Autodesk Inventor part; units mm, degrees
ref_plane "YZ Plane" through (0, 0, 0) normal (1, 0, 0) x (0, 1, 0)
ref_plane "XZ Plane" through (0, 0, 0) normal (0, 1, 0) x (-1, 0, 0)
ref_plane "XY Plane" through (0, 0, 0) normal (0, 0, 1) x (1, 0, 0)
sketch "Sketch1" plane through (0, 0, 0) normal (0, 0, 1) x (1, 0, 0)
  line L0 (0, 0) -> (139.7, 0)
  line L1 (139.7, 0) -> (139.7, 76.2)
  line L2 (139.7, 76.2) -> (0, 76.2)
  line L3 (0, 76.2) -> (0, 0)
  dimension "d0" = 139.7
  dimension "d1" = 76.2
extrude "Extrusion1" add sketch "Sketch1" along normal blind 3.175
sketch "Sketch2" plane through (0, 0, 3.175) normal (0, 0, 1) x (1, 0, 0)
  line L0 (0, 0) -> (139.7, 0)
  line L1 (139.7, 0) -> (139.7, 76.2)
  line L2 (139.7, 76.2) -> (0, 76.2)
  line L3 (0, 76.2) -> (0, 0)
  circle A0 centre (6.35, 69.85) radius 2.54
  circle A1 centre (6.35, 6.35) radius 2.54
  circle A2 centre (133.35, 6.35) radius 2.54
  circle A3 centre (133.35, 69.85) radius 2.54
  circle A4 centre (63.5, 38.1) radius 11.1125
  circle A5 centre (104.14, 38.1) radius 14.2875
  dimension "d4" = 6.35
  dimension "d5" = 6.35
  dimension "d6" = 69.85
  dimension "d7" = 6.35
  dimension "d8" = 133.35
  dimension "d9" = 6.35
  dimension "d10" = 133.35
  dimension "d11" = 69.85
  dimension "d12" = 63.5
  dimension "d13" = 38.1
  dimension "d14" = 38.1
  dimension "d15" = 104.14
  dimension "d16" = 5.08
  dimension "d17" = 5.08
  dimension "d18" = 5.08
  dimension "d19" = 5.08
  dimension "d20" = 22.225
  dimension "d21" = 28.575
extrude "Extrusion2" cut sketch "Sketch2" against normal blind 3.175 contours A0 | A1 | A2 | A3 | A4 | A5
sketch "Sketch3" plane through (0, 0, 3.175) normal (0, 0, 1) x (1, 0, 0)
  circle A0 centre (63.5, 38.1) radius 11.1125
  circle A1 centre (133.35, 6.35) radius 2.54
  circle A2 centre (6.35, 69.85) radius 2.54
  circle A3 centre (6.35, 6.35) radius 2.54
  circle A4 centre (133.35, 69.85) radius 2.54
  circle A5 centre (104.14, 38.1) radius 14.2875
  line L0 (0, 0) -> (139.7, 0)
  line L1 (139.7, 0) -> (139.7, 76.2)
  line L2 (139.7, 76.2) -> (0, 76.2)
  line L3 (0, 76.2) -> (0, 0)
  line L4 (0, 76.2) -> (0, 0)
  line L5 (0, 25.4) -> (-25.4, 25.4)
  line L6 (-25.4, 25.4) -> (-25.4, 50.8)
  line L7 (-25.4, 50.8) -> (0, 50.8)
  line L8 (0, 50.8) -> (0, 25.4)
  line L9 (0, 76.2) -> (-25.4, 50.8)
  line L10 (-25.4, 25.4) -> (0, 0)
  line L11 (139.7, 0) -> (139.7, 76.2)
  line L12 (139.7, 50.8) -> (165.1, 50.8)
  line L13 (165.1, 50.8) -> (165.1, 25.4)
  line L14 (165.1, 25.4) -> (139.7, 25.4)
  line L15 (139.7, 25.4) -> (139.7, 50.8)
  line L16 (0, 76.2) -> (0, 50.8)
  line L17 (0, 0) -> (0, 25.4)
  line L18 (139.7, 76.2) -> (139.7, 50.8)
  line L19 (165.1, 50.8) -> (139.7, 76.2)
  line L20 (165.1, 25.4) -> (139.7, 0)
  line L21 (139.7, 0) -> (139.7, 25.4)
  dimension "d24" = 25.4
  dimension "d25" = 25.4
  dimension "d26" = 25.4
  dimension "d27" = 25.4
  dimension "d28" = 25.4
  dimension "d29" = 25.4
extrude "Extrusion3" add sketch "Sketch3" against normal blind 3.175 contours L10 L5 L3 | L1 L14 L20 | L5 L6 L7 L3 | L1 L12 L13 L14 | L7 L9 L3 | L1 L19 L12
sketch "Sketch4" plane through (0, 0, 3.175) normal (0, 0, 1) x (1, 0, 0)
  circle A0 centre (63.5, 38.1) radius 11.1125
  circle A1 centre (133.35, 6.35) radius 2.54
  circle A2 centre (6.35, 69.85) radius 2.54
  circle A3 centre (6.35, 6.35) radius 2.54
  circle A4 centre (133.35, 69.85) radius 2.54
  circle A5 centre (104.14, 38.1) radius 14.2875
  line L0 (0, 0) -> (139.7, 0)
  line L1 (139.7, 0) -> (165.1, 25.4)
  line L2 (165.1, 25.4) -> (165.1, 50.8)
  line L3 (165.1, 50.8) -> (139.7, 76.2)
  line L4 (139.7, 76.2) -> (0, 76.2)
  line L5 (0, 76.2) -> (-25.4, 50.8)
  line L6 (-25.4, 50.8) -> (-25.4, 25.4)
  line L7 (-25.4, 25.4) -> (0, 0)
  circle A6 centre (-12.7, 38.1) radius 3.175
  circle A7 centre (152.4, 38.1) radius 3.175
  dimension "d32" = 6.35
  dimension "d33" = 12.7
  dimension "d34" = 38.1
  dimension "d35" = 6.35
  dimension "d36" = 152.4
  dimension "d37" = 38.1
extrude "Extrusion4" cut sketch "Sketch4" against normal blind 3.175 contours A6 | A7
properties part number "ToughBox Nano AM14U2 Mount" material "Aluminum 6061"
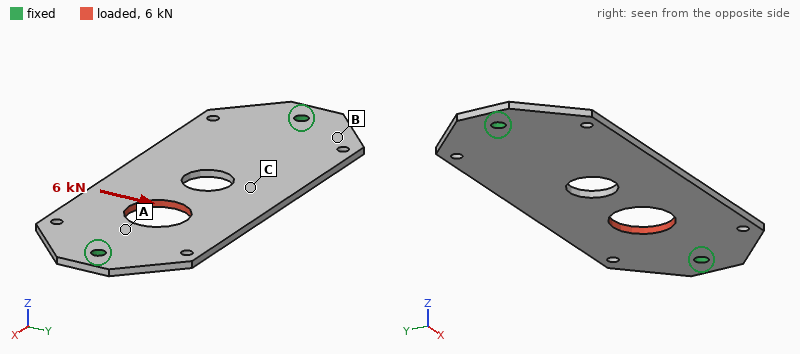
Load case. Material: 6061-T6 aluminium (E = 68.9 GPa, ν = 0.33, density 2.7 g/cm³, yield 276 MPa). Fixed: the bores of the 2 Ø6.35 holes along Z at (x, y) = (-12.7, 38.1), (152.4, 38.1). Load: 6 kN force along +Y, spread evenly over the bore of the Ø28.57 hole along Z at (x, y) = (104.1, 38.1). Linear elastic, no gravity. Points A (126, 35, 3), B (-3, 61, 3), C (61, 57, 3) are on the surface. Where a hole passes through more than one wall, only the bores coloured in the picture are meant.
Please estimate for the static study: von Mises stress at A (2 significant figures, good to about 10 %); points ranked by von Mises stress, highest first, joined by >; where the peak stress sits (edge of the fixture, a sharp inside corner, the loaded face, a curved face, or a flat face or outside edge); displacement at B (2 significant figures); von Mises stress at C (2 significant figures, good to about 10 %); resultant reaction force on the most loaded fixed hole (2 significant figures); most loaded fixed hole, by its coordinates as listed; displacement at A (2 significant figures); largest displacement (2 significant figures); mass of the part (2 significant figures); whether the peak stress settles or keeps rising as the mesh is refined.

48 MPa
A > C > B
edge of the fixture
24 µm
29 MPa
4.3 kN
(152.4, 38.1)
55 µm
100 µm
100 g
keeps rising
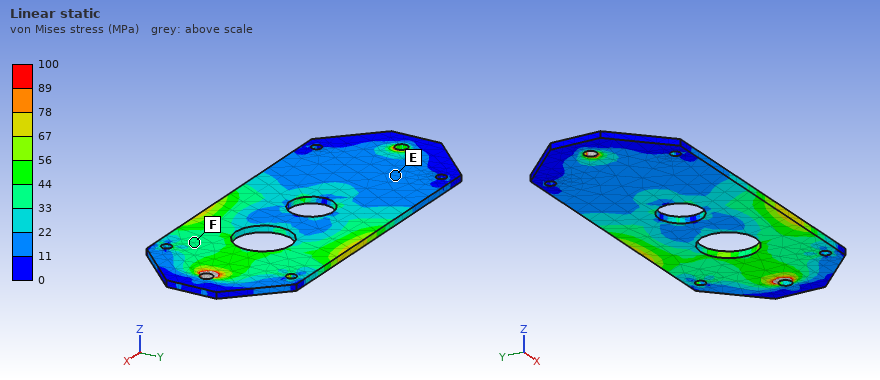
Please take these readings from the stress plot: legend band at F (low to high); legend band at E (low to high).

33 to 44 MPa
11 to 22 MPa
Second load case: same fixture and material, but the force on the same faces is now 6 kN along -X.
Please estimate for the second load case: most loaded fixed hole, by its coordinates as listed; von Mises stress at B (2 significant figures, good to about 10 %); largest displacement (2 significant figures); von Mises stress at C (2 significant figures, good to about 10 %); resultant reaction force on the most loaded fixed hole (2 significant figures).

(152.4, 38.1)
6.5 MPa
33 µm
17 MPa
3.8 kN
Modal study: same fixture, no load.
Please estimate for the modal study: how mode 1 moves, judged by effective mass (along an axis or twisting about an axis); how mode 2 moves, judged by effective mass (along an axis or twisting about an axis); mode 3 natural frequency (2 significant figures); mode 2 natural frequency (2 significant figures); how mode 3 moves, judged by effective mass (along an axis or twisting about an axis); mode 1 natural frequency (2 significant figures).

along Z
twisting about X
1400 Hz
680 Hz
twisting about Y
540 Hz
